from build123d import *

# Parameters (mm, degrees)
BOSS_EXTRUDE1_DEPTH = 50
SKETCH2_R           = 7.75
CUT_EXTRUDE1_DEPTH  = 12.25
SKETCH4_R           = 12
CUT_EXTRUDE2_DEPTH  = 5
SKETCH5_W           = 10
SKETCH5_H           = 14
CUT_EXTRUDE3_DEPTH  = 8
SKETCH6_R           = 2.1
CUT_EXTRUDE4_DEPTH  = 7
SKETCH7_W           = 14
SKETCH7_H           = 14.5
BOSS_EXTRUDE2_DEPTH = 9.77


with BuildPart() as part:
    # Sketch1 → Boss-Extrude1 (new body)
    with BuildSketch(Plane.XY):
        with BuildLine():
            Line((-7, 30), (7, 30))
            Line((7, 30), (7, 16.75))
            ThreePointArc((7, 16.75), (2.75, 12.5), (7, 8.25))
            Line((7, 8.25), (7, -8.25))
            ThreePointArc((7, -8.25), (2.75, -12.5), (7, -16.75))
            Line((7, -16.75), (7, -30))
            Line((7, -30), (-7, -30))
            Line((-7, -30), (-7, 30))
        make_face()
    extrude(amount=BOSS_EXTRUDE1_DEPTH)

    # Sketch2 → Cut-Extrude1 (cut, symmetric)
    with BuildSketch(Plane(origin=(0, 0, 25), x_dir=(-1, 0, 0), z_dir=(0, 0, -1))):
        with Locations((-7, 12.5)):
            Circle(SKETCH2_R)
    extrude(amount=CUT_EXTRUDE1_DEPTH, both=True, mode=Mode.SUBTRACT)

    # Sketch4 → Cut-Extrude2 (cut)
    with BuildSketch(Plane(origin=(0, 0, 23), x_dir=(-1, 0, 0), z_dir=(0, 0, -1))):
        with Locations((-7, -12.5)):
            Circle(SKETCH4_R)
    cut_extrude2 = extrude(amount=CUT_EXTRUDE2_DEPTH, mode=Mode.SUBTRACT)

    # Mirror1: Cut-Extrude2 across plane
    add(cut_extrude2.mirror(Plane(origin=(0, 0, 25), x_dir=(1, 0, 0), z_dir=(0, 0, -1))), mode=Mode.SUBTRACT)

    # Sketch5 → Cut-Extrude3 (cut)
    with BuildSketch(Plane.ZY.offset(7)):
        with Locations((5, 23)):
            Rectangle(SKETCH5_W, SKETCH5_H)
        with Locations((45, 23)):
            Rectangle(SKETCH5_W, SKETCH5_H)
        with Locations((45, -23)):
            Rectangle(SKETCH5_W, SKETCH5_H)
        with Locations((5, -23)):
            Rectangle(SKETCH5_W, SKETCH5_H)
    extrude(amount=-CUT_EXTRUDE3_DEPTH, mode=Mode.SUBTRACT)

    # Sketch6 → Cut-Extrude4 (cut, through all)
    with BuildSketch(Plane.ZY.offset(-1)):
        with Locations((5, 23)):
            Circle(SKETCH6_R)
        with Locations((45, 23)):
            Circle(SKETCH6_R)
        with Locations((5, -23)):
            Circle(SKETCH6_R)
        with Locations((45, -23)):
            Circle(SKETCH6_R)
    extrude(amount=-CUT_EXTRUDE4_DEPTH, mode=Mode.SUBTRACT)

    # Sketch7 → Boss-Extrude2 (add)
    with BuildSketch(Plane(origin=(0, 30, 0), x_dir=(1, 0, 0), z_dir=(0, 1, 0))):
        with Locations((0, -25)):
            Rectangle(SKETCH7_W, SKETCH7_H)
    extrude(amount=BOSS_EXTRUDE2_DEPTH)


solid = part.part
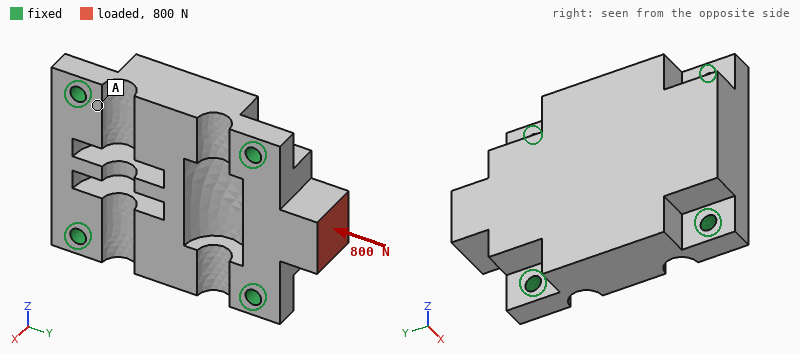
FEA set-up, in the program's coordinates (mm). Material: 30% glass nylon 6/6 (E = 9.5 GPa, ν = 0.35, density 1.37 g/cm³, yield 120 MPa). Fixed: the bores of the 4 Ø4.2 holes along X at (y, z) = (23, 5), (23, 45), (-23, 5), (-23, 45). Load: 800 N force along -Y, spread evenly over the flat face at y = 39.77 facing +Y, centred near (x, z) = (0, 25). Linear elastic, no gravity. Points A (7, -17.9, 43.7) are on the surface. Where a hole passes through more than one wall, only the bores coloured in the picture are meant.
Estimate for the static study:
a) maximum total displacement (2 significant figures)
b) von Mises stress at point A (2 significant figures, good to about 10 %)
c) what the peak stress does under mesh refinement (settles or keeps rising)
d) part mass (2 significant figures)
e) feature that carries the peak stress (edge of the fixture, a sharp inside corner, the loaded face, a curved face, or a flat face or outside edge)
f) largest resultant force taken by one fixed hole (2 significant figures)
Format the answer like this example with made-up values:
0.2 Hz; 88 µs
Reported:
20 µm; 0.95 MPa; keeps rising; 45 g; edge of the fixture; 260 N
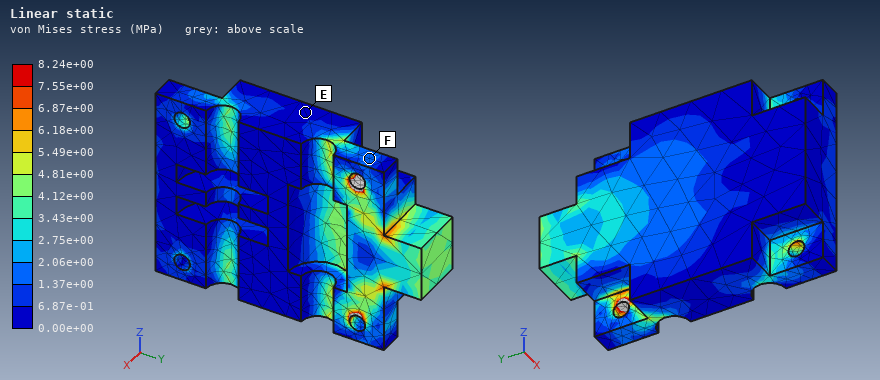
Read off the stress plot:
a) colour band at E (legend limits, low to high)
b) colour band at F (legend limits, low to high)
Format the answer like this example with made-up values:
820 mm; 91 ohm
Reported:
0.00e+00 to 6.87e-01 MPa; 1.37e+00 to 2.06e+00 MPa
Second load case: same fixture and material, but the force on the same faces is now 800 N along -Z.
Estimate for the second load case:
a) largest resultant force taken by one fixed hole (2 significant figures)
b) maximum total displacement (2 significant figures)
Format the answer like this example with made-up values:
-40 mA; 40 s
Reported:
490 N; 55 µm
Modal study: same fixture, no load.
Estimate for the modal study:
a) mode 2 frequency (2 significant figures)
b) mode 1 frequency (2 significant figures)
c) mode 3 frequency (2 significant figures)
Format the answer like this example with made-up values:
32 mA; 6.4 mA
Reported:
7100 Hz; 7000 Hz; 8600 Hz
